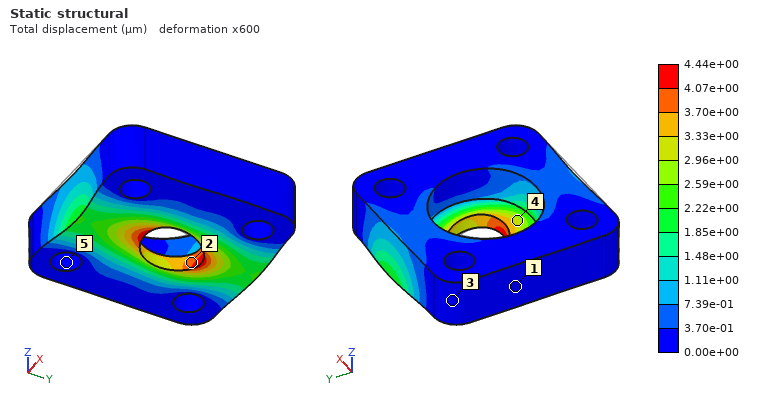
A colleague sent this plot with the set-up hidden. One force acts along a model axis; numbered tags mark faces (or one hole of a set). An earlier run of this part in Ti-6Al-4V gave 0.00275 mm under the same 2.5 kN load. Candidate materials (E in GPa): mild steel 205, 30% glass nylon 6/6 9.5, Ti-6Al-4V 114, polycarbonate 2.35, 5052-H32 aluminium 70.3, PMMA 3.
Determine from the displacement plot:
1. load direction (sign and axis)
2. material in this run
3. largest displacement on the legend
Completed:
+Y
5052-H32 aluminium
4.44e+00 µm
